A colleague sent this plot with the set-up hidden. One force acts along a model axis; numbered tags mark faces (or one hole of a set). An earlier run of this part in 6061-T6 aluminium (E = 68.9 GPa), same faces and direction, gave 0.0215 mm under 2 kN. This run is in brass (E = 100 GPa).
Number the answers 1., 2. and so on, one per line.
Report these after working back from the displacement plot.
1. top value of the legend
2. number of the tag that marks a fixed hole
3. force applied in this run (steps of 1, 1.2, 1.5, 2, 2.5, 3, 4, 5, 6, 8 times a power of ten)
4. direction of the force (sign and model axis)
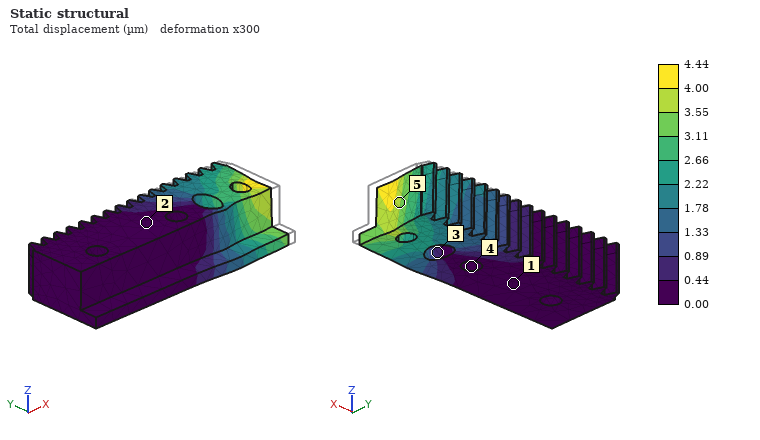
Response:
1. 4.44 µm
2. 4
3. 600 N
4. -X
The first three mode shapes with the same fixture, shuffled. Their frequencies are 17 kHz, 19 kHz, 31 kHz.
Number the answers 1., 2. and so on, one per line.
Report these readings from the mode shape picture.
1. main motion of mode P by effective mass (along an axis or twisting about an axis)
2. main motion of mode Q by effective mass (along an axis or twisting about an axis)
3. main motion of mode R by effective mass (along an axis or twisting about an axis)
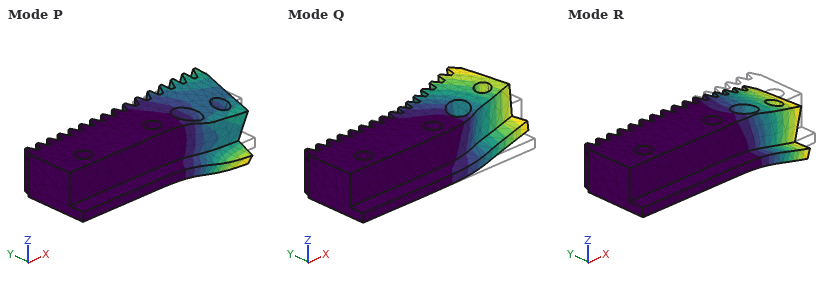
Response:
1. twisting about X
2. along Y
3. along Z
